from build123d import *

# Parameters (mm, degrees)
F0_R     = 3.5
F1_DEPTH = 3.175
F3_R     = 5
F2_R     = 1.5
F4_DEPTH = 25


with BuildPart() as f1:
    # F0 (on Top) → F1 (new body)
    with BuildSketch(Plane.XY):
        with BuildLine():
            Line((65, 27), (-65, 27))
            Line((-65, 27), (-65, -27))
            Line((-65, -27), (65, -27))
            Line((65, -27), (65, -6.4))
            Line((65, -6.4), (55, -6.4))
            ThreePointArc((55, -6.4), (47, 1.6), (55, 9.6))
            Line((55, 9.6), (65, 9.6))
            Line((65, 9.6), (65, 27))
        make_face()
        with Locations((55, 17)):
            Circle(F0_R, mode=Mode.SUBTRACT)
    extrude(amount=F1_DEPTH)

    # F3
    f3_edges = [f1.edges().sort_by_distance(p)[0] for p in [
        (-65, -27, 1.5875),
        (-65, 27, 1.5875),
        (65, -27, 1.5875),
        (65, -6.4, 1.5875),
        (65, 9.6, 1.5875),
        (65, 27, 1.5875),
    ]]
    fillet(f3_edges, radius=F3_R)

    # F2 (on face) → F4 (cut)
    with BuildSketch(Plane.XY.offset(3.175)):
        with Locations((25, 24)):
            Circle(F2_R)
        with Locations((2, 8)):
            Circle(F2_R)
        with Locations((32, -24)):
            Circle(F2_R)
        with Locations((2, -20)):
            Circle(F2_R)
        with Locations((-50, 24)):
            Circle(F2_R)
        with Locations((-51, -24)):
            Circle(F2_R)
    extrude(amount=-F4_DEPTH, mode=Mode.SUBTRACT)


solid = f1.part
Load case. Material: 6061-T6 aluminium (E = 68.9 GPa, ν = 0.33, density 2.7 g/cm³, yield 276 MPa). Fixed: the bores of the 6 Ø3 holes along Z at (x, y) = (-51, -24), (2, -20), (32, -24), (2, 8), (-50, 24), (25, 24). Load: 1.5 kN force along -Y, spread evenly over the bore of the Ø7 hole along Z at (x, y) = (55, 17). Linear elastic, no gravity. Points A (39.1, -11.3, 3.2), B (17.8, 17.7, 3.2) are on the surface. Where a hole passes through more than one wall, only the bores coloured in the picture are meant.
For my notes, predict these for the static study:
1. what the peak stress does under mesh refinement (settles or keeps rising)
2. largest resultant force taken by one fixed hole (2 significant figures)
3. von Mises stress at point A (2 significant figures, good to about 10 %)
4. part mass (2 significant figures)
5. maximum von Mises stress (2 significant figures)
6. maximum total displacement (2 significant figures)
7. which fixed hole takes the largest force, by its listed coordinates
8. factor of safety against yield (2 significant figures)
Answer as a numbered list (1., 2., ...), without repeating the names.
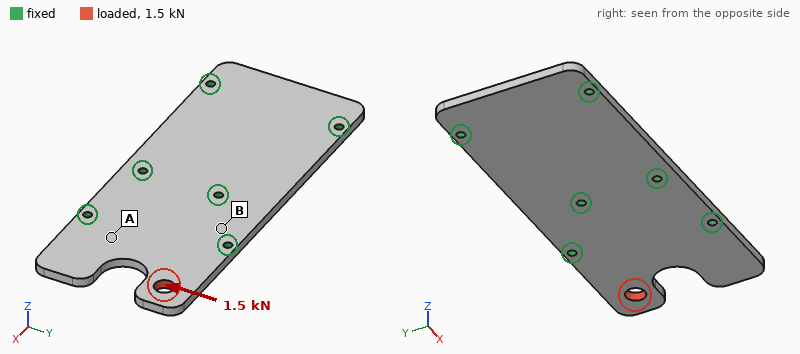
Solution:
1. settles
2. 1.1 kN
3. 23 MPa
4. 57 g
5. 140 MPa
6. 68 µm
7. (25, 24)
8. 2.0
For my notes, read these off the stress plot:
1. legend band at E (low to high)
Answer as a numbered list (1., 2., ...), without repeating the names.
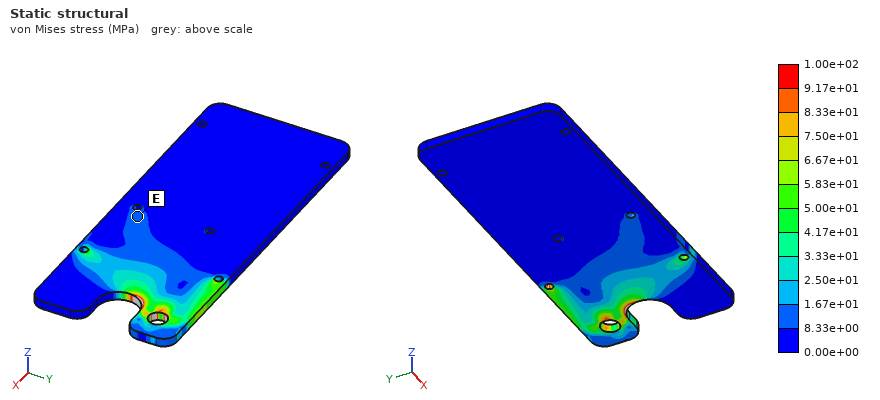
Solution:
1. 8.33e+00 to 1.67e+01 MPa
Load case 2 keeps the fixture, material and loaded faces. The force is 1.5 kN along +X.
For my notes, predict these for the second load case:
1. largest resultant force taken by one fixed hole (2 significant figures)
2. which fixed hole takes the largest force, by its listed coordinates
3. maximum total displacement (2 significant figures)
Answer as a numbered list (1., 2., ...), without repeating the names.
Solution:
1. 990 N
2. (25, 24)
3. 16 µm
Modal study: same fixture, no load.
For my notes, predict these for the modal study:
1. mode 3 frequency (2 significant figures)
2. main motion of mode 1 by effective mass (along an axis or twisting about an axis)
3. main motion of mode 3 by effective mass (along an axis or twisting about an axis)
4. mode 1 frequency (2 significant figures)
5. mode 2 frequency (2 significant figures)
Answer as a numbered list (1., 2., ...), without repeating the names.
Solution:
1. 4700 Hz
2. along Z
3. along Z
4. 2000 Hz
5. 2900 Hz
